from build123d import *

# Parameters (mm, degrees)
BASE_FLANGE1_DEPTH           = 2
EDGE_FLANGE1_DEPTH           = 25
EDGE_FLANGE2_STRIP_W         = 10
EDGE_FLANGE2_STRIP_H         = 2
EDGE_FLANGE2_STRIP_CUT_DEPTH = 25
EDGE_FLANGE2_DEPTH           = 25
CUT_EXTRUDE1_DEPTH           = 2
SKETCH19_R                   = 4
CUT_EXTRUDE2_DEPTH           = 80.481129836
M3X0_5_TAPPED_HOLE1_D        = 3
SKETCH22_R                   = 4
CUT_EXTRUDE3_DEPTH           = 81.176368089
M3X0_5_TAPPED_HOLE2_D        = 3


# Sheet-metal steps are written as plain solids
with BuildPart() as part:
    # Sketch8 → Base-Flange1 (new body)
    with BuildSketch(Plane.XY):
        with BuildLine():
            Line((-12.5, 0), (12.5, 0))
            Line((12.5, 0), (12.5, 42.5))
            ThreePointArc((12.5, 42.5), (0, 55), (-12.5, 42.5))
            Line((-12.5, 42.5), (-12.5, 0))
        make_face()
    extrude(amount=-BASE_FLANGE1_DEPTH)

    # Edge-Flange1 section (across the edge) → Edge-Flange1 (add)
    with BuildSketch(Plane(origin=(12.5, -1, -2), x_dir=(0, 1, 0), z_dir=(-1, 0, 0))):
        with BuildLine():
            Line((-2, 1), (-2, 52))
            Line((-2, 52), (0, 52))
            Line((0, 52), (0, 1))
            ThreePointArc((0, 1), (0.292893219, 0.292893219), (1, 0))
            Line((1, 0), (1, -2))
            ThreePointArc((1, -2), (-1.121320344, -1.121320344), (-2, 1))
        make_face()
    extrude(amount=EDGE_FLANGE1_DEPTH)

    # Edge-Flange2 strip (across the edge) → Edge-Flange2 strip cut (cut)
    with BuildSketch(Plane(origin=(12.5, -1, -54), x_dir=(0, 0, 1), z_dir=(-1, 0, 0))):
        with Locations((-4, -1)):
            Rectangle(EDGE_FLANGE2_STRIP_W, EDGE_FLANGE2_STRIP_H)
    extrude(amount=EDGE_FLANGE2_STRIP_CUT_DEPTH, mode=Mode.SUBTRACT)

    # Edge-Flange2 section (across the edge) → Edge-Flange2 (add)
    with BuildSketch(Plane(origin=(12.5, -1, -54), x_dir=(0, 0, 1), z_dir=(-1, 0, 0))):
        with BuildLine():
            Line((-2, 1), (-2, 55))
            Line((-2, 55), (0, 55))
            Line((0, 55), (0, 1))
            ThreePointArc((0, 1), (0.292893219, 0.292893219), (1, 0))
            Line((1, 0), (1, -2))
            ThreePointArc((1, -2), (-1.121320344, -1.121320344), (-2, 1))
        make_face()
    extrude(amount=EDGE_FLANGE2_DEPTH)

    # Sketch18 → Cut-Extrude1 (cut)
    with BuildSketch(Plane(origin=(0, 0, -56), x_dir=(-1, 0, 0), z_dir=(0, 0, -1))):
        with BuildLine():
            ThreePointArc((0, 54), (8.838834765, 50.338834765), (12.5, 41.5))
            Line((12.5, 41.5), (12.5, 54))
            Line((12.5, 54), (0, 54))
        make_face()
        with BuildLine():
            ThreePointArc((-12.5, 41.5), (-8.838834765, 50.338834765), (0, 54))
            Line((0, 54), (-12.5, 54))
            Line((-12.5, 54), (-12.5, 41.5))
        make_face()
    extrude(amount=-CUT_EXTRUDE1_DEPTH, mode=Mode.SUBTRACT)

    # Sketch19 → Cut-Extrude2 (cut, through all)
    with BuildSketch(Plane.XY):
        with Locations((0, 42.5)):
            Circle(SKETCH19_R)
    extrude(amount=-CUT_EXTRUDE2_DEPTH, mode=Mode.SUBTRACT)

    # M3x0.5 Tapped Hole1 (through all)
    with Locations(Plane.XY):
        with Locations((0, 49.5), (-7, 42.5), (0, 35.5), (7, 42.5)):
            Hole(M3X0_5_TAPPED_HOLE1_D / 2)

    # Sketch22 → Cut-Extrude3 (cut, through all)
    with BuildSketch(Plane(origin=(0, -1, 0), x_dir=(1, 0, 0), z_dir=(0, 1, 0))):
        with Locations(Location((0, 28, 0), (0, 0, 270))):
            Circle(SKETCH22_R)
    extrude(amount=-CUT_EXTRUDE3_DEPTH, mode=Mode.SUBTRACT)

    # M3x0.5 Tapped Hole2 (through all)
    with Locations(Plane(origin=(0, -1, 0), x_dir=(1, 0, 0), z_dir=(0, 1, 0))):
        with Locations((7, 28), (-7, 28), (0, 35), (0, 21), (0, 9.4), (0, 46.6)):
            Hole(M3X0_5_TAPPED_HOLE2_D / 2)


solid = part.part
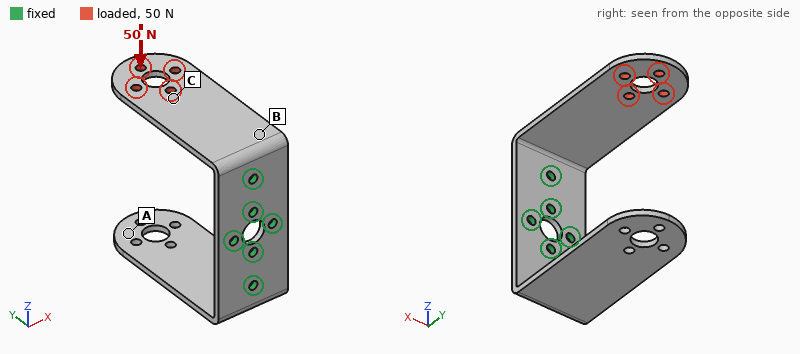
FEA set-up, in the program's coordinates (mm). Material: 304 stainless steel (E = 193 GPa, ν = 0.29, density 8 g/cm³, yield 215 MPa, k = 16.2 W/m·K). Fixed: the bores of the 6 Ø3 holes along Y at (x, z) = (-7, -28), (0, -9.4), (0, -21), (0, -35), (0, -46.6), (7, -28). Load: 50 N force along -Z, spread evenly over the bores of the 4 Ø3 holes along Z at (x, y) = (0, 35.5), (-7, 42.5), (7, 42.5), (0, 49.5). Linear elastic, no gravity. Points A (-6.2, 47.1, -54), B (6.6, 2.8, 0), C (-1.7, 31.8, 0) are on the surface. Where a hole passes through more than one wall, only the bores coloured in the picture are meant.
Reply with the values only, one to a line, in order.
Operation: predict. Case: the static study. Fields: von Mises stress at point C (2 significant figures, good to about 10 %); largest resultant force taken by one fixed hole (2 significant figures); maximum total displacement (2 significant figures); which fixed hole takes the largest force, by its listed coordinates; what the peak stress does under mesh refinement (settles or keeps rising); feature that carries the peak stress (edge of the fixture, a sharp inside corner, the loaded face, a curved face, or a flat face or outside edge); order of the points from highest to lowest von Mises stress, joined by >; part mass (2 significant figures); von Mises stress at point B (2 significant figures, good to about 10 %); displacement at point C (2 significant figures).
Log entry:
33 MPa
90 N
0.95 mm
(0, -9.4)
keeps rising
edge of the fixture
B > C > A
60 g
110 MPa
0.47 mm
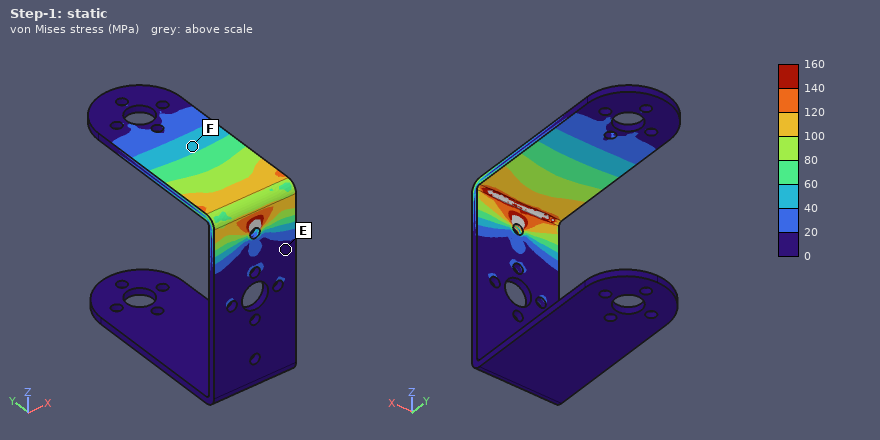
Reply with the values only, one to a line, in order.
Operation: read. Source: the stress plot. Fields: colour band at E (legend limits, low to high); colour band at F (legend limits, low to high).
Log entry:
0 to 20 MPa
40 to 60 MPa
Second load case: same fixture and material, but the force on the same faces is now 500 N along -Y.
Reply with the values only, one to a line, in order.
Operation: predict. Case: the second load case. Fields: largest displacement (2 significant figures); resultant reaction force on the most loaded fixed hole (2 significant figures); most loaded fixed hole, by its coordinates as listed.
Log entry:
0.35 mm
610 N
(0, -9.4)
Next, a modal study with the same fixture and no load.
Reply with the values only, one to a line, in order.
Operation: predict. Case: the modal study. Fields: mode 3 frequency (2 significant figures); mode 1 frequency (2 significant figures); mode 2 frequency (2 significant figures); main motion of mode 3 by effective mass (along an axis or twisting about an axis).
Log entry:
910 Hz
460 Hz
480 Hz
along X
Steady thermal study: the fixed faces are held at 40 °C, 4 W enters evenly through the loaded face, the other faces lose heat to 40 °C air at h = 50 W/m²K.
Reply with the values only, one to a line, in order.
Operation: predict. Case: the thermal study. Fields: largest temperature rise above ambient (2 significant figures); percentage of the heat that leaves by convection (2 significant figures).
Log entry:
63 K
94 %
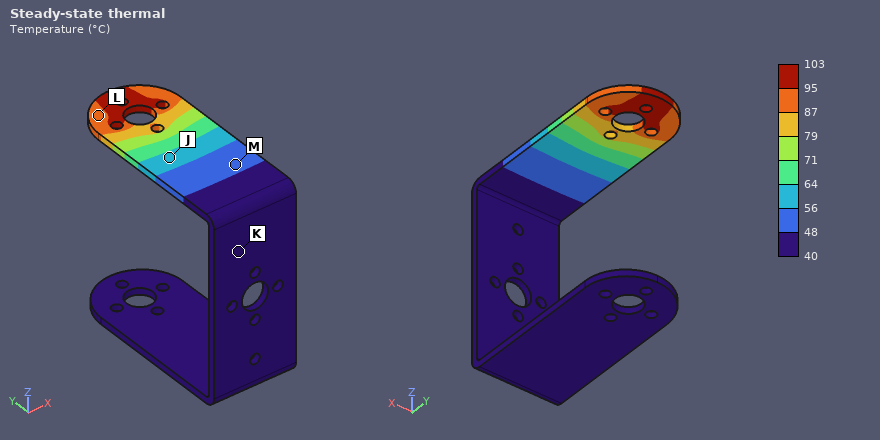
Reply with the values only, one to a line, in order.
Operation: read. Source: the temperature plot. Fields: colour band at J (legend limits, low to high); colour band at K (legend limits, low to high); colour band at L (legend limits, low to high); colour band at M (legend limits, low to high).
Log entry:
56 to 64 °C
40 to 48 °C
87 to 95 °C
48 to 56 °C
